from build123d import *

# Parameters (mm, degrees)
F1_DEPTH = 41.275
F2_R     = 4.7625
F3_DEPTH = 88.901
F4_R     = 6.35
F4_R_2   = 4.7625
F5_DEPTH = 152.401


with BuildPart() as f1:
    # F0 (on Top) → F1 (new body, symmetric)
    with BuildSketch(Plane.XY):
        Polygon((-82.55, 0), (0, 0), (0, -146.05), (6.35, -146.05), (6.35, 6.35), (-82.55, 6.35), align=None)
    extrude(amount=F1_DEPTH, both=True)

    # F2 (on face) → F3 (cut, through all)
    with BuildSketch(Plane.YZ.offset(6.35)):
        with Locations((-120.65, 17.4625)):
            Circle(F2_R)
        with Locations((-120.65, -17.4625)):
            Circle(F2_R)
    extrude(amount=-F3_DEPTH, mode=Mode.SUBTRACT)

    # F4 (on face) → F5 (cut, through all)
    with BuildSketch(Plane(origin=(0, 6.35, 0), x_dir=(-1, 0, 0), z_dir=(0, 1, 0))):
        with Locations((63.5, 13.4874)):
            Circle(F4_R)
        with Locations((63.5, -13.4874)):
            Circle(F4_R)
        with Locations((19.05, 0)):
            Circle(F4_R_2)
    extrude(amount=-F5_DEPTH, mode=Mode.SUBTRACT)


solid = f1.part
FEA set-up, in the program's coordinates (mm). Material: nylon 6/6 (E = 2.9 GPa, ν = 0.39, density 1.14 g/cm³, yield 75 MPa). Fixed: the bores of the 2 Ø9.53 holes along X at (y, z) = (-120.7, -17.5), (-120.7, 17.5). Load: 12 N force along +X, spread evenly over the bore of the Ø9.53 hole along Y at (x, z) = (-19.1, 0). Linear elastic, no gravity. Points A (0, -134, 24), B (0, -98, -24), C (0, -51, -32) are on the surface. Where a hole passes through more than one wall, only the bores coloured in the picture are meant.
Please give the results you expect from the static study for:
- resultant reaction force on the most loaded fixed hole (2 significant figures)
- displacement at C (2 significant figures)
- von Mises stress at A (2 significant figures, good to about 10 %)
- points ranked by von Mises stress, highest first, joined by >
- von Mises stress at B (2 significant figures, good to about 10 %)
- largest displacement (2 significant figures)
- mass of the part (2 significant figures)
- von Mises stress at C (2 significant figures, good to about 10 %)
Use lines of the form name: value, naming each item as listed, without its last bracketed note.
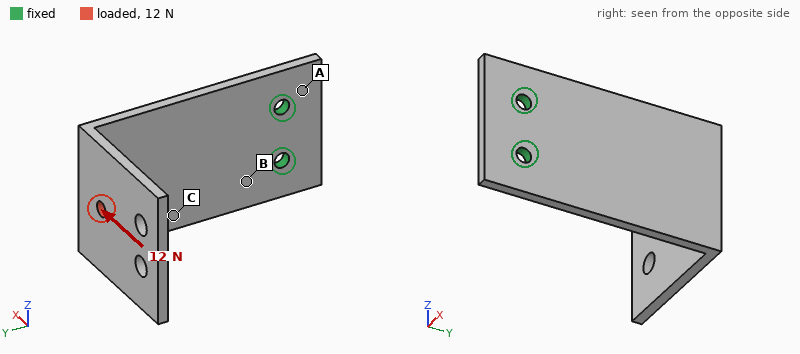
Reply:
resultant reaction force on the most loaded fixed hole: 6.0 N
displacement at C: 0.50 mm
von Mises stress at A: 0.39 MPa
points ranked by von Mises stress, highest first, joined by >: B > C > A
von Mises stress at B: 2.0 MPa
largest displacement: 2.0 mm
mass of the part: 140 g
von Mises stress at C: 1.2 MPa
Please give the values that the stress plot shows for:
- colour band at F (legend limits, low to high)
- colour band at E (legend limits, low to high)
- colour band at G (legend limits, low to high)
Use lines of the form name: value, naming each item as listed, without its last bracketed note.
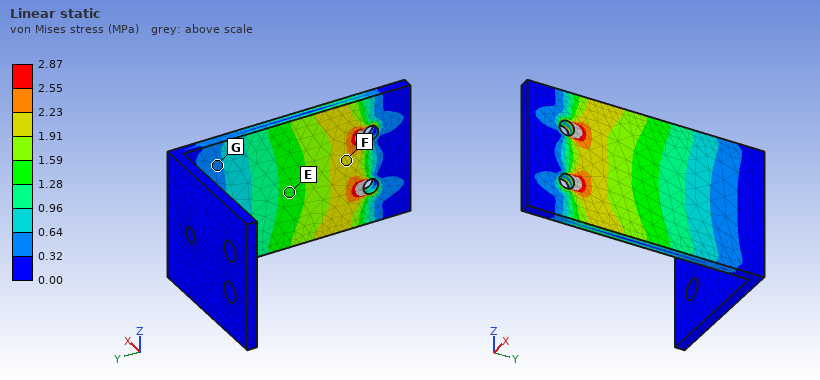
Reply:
colour band at F: 1.91 to 2.23 MPa
colour band at E: 1.28 to 1.59 MPa
colour band at G: 0.32 to 0.64 MPa
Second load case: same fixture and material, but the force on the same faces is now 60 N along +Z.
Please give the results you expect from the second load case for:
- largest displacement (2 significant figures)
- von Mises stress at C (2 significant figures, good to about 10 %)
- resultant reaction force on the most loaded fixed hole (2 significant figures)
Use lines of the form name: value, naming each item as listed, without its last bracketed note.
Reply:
largest displacement: 1.8 mm
von Mises stress at C: 2.1 MPa
resultant reaction force on the most loaded fixed hole: 180 N
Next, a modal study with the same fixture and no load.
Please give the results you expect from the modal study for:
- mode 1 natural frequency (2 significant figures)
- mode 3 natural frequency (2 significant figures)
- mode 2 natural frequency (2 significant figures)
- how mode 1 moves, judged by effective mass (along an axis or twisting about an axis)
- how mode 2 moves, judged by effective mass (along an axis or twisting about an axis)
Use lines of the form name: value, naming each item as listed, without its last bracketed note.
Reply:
mode 1 natural frequency: 51 Hz
mode 3 natural frequency: 170 Hz
mode 2 natural frequency: 110 Hz
how mode 1 moves, judged by effective mass: along X
how mode 2 moves, judged by effective mass: along Z
